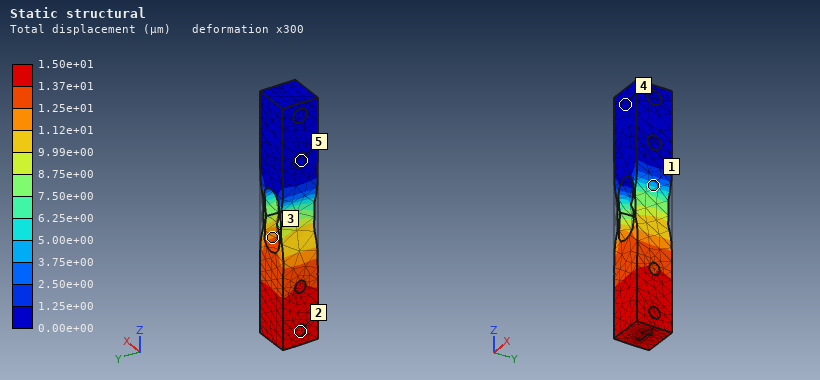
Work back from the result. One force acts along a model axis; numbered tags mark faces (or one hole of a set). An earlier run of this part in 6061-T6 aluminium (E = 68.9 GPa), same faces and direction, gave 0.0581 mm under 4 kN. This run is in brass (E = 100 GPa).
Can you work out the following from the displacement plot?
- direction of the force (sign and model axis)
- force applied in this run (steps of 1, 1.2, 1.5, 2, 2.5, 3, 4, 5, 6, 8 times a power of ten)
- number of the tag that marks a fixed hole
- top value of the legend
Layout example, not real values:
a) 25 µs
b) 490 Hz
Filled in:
a) -Z
b) 1.5 kN
c) 5
d) 1.50e+01 µm
